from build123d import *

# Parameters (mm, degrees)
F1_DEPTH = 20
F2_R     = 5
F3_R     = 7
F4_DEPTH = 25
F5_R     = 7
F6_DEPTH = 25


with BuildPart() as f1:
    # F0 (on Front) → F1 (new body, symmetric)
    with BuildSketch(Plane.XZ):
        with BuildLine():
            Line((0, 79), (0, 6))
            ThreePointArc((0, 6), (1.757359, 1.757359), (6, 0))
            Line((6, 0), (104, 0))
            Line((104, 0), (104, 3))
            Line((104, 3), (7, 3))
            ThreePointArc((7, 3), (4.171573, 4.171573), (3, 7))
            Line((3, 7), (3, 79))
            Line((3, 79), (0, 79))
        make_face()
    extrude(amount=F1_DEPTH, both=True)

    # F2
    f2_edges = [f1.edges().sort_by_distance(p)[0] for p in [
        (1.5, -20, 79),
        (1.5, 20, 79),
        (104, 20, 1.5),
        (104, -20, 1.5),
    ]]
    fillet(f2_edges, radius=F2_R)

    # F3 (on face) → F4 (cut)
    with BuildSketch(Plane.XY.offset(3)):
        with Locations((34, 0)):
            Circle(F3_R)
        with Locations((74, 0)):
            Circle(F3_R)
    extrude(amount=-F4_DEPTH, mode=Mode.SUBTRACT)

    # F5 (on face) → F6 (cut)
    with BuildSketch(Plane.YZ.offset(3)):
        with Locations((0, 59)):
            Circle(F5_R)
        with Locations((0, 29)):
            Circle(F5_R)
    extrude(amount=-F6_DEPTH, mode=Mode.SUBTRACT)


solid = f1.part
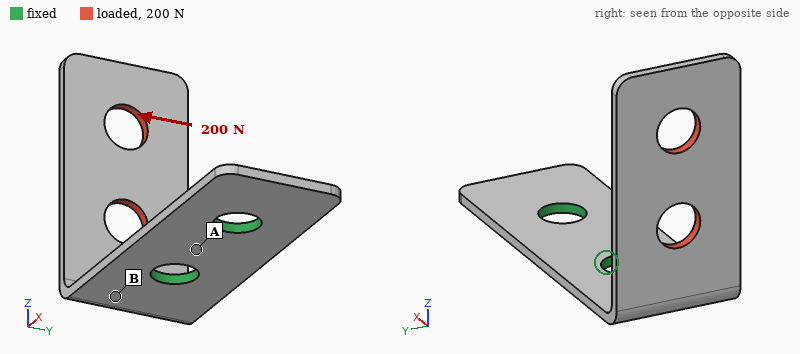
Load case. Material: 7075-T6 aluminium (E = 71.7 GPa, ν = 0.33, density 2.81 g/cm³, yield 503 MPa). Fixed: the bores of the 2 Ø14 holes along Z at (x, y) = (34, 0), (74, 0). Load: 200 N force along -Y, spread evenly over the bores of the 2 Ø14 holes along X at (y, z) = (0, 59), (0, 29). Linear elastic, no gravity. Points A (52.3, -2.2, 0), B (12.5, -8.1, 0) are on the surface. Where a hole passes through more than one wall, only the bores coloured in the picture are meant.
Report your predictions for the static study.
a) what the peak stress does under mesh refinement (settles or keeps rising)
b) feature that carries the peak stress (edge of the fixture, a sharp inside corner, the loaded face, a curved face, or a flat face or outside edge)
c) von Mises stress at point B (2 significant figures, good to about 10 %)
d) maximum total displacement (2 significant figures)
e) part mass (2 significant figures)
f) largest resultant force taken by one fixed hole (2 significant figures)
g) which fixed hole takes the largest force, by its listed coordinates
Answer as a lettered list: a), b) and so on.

a) keeps rising
b) edge of the fixture
c) 83 MPa
d) 1.4 mm
e) 55 g
f) 260 N
g) (34, 0)
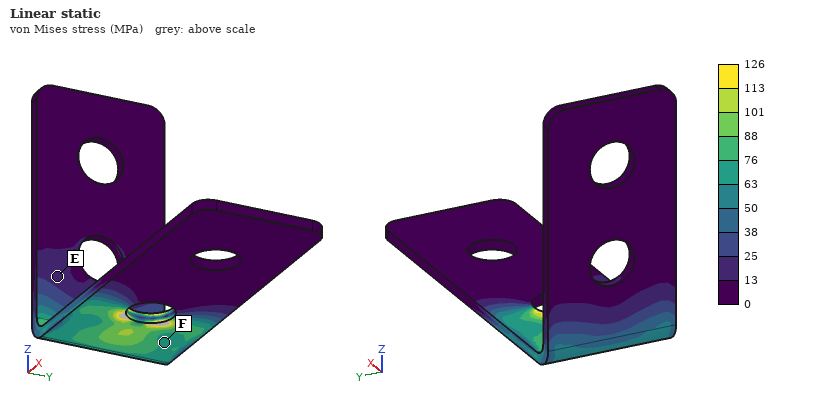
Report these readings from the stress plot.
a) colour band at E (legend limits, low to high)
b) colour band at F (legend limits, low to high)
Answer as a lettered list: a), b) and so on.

a) 13 to 25 MPa
b) 63 to 76 MPa
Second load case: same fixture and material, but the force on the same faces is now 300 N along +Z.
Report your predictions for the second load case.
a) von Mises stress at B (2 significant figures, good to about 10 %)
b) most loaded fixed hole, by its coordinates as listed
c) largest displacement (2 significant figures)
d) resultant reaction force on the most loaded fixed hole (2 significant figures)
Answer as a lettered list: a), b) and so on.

a) 50 MPa
b) (34, 0)
c) 1.3 mm
d) 310 N
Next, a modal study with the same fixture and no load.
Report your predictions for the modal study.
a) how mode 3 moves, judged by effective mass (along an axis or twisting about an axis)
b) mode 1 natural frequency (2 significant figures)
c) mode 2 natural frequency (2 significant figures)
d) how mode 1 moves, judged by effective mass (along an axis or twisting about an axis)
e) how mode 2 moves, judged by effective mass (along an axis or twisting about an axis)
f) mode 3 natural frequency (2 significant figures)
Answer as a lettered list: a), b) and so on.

a) along Z
b) 280 Hz
c) 500 Hz
d) along X
e) along Y
f) 1200 Hz
